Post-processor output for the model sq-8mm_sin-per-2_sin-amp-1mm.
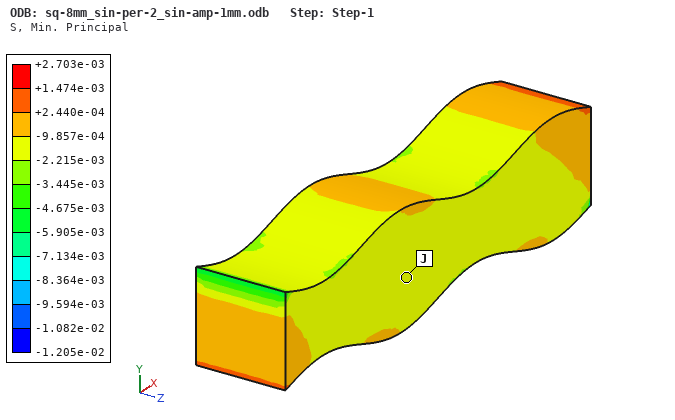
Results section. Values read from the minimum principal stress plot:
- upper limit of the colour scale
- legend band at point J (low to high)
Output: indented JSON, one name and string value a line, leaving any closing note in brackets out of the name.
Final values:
{
  "upper limit of the colour scale": "+2.703e-03",
  "legend band at point J": "-2.215e-03 to -9.857e-04"
}
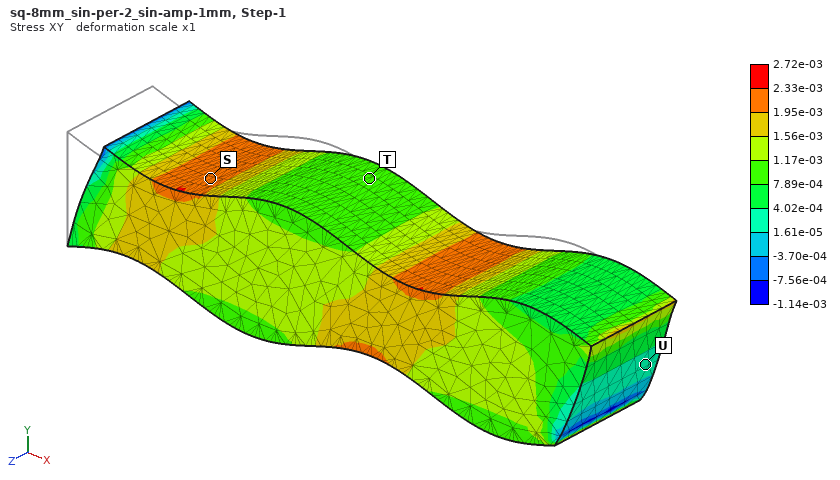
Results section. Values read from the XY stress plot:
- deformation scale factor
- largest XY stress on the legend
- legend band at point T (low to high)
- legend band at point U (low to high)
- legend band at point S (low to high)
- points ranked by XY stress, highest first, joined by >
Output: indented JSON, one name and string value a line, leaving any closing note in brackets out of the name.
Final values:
{
  "deformation scale factor": "1",
  "largest XY stress on the legend": "2.72e-03",
  "legend band at point T": "7.89e-04 to 1.17e-03",
  "legend band at point U": "1.61e-05 to 4.02e-04",
  "legend band at point S": "1.95e-03 to 2.33e-03",
  "points ranked by XY stress, highest first, joined by >": "S > T > U"
}
